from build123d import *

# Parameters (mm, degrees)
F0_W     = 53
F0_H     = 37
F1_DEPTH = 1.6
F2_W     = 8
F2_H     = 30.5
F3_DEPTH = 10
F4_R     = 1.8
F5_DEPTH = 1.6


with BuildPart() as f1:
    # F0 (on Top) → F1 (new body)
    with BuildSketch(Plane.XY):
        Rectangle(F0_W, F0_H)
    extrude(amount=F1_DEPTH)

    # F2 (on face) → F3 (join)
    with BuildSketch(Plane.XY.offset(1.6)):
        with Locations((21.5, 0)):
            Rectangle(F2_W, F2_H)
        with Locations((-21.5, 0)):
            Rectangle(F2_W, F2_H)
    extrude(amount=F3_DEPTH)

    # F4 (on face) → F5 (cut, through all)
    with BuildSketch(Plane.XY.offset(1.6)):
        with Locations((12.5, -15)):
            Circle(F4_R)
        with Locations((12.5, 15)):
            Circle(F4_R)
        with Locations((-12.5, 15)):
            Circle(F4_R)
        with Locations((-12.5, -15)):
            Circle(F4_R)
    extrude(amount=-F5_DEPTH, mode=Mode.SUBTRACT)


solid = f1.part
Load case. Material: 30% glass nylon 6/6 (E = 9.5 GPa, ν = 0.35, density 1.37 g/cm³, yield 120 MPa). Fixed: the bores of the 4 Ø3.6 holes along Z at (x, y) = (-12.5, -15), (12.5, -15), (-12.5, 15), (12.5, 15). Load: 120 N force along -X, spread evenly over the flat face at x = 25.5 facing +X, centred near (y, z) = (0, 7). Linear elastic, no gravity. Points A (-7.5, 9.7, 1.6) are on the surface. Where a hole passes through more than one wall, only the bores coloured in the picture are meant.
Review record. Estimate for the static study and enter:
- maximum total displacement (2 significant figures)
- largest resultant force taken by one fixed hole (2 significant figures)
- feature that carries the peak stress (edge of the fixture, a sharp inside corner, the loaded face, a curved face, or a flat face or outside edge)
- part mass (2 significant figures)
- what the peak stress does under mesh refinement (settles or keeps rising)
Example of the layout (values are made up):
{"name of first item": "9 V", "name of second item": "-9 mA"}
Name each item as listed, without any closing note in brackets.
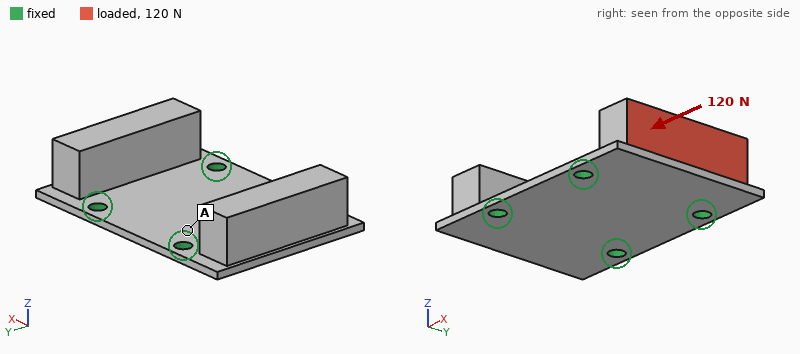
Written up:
{"maximum total displacement": "0.45 mm", "largest resultant force taken by one fixed hole": "46 N", "feature that carries the peak stress": "edge of the fixture", "part mass": "11 g", "what the peak stress does under mesh refinement": "keeps rising"}
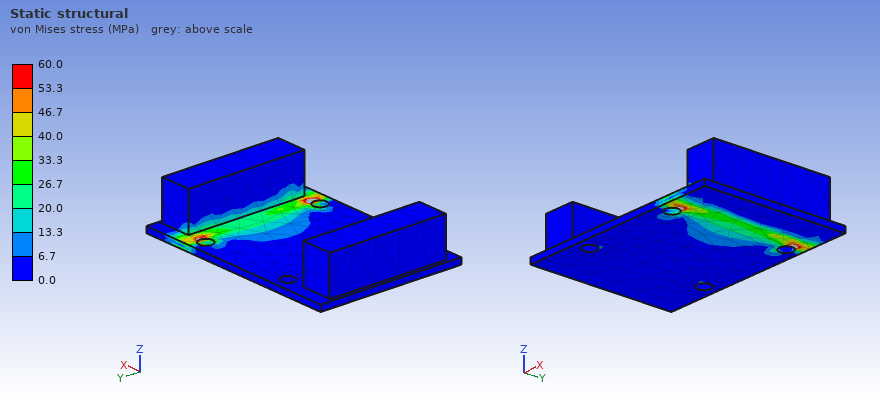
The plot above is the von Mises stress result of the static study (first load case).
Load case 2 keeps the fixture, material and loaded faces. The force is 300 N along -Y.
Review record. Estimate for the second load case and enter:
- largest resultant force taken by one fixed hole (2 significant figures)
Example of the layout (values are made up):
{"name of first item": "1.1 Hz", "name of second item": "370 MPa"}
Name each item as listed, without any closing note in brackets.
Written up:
{"largest resultant force taken by one fixed hole": "200 N"}
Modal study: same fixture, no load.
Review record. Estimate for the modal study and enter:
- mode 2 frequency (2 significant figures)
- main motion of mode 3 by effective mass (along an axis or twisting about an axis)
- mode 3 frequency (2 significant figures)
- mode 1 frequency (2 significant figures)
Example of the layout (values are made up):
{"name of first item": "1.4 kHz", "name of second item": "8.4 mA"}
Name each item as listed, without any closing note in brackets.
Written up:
{"mode 2 frequency": "1400 Hz", "main motion of mode 3 by effective mass": "along Z", "mode 3 frequency": "5200 Hz", "mode 1 frequency": "1300 Hz"}
